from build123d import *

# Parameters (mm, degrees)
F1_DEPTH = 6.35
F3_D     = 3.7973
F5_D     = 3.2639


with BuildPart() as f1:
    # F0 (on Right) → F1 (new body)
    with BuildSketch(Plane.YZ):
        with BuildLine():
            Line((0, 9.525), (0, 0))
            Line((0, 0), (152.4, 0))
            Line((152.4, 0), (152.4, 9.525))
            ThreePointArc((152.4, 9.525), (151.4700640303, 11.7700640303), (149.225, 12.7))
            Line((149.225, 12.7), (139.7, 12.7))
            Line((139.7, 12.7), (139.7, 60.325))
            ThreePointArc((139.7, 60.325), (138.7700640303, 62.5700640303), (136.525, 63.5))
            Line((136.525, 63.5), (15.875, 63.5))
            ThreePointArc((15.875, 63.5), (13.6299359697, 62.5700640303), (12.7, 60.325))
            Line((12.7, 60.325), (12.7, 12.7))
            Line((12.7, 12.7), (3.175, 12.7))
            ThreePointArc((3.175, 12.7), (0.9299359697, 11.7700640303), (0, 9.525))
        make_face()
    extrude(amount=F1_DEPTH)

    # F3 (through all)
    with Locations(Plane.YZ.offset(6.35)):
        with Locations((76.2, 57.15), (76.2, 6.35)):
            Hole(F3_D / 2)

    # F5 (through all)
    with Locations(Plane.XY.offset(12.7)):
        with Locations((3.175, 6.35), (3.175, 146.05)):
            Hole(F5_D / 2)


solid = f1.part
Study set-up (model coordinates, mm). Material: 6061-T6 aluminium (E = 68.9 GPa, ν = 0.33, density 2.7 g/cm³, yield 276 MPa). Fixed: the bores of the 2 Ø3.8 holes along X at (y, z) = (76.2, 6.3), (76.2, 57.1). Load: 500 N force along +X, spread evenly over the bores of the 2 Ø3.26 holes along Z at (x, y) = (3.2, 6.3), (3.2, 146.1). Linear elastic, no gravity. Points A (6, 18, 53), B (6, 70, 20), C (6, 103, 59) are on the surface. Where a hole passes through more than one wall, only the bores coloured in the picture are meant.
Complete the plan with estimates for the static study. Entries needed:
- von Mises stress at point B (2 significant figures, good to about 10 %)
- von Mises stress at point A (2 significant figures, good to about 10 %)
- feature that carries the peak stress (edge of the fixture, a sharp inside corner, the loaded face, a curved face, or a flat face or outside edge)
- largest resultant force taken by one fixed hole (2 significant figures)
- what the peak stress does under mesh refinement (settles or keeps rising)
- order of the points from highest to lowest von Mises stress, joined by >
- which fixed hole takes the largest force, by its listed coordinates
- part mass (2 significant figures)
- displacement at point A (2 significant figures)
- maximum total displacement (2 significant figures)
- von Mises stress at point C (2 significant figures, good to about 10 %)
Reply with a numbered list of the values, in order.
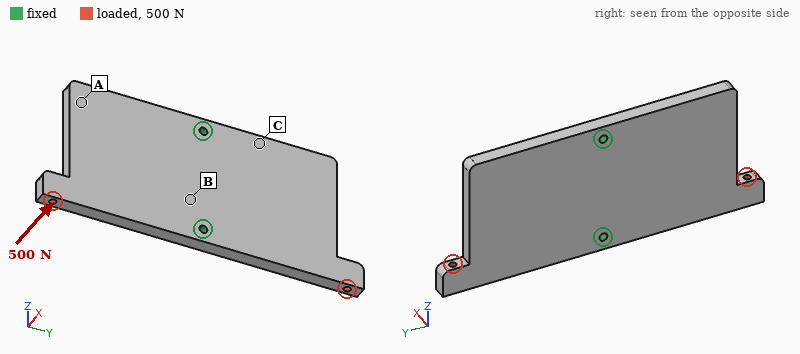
1. 39 MPa
2. 7.7 MPa
3. edge of the fixture
4. 500 N
5. keeps rising
6. B > C > A
7. (76.2, 6.3)
8. 140 g
9. 0.17 mm
10. 0.45 mm
11. 22 MPa
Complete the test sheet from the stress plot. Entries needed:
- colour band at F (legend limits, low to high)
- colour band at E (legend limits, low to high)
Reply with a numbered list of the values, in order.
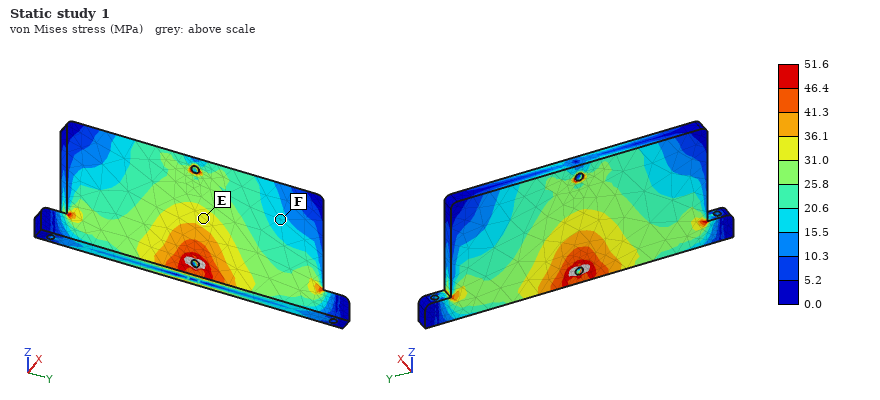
1. 15.5 to 20.6 MPa
2. 31.0 to 36.1 MPa
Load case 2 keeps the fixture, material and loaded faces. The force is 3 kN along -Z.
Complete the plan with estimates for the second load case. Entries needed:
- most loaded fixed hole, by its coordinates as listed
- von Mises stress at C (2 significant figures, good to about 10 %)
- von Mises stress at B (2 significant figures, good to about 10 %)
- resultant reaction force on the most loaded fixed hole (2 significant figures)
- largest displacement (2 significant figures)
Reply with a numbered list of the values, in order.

1. (76.2, 57.1)
2. 11 MPa
3. 7.8 MPa
4. 1.6 kN
5. 78 µm
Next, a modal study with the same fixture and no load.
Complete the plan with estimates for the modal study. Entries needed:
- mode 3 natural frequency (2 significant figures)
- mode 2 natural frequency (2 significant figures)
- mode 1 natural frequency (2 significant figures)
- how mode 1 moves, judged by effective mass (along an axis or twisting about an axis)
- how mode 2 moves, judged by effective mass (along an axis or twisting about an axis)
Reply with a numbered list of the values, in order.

1. 2700 Hz
2. 1200 Hz
3. 920 Hz
4. twisting about Z
5. along X
